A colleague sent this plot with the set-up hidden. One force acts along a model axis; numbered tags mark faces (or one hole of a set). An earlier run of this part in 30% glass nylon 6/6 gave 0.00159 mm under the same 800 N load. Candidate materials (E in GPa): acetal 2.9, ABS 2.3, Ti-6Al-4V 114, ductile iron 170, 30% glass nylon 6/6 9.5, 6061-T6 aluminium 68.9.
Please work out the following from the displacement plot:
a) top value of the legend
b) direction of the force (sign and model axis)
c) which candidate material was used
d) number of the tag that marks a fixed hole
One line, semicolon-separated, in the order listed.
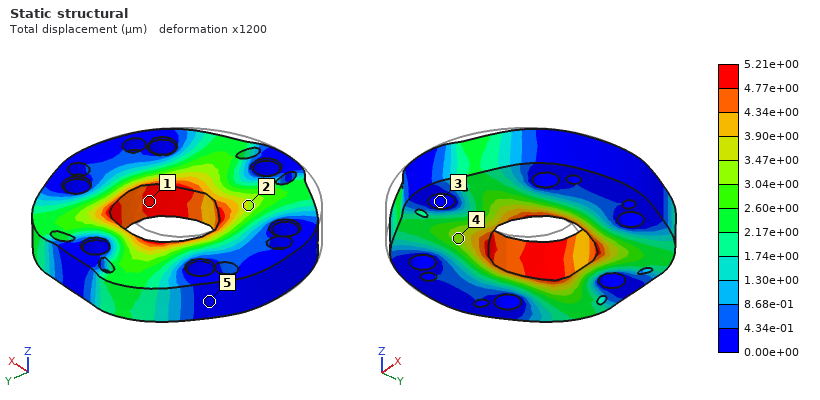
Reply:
5.21e+00 µm; +Y; acetal; 3
